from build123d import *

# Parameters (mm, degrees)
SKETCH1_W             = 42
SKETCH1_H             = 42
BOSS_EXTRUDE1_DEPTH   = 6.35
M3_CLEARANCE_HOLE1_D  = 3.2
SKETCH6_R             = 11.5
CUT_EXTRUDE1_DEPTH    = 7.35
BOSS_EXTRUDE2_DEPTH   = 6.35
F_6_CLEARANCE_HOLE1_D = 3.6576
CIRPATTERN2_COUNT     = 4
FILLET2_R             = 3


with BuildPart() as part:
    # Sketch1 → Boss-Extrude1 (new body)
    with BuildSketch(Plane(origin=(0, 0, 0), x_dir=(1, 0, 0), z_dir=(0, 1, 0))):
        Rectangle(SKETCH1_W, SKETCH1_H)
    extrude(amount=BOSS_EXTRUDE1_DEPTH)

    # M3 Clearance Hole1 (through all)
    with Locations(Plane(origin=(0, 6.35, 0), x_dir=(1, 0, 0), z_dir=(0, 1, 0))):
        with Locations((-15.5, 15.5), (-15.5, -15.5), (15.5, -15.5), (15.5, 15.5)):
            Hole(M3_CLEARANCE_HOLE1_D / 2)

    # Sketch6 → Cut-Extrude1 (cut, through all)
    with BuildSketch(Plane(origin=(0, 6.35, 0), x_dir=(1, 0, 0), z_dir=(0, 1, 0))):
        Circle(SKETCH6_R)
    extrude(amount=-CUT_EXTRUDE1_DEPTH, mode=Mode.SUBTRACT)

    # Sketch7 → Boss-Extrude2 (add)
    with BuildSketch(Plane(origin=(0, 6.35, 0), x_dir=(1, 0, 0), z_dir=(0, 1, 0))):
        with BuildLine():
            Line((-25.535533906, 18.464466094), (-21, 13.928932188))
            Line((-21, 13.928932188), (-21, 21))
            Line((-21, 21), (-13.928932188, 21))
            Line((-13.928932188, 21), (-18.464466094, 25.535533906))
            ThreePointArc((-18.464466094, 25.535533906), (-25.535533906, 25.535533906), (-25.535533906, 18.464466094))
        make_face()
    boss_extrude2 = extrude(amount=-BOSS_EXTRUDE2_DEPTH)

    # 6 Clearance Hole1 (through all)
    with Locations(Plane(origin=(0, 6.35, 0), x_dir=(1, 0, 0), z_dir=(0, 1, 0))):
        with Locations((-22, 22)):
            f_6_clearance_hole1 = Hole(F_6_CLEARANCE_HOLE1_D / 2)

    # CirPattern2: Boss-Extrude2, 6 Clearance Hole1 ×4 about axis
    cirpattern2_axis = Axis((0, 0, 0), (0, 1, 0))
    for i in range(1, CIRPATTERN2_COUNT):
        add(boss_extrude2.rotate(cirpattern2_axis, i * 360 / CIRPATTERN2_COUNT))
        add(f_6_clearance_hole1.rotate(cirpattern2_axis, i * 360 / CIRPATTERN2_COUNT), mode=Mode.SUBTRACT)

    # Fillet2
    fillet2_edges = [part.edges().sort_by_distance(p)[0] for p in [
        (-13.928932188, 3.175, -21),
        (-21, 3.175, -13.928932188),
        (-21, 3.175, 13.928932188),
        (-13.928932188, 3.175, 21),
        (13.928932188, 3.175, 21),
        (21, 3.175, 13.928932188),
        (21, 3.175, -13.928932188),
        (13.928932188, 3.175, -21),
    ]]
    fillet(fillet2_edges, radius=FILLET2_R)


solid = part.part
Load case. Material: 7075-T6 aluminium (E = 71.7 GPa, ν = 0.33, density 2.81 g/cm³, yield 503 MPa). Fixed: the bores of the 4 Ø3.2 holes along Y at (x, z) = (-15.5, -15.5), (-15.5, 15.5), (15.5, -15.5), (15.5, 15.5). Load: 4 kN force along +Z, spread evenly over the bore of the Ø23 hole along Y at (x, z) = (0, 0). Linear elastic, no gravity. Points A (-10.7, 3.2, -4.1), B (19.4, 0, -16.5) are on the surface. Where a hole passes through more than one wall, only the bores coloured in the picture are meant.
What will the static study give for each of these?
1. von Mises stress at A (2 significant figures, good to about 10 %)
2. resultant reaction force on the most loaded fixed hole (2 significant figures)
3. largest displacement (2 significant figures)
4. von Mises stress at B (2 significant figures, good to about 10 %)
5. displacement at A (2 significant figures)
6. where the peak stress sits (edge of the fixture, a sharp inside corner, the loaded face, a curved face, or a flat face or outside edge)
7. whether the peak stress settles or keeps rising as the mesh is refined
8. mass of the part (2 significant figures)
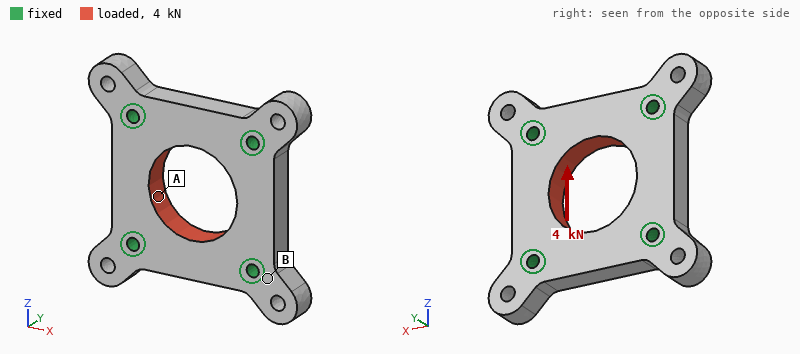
19 MPa
1.0 kN
5.8 µm
6.6 MPa
2.5 µm
edge of the fixture
keeps rising
28 g
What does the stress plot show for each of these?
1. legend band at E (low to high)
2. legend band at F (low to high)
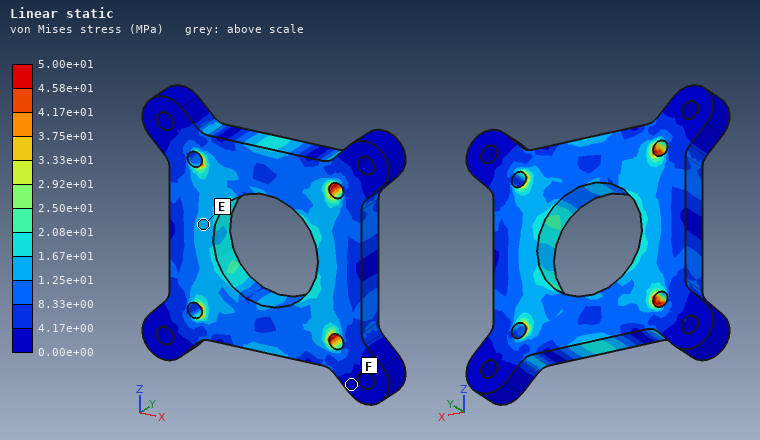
1.25e+01 to 1.67e+01 MPa
0.00e+00 to 4.17e+00 MPa
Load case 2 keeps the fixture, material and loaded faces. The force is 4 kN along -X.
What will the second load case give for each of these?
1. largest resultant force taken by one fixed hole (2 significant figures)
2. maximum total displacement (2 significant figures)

1.0 kN
5.9 µm
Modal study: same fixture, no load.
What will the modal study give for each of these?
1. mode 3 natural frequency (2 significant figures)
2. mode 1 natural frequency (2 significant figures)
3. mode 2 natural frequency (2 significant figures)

27 kHz
24 kHz
26 kHz
